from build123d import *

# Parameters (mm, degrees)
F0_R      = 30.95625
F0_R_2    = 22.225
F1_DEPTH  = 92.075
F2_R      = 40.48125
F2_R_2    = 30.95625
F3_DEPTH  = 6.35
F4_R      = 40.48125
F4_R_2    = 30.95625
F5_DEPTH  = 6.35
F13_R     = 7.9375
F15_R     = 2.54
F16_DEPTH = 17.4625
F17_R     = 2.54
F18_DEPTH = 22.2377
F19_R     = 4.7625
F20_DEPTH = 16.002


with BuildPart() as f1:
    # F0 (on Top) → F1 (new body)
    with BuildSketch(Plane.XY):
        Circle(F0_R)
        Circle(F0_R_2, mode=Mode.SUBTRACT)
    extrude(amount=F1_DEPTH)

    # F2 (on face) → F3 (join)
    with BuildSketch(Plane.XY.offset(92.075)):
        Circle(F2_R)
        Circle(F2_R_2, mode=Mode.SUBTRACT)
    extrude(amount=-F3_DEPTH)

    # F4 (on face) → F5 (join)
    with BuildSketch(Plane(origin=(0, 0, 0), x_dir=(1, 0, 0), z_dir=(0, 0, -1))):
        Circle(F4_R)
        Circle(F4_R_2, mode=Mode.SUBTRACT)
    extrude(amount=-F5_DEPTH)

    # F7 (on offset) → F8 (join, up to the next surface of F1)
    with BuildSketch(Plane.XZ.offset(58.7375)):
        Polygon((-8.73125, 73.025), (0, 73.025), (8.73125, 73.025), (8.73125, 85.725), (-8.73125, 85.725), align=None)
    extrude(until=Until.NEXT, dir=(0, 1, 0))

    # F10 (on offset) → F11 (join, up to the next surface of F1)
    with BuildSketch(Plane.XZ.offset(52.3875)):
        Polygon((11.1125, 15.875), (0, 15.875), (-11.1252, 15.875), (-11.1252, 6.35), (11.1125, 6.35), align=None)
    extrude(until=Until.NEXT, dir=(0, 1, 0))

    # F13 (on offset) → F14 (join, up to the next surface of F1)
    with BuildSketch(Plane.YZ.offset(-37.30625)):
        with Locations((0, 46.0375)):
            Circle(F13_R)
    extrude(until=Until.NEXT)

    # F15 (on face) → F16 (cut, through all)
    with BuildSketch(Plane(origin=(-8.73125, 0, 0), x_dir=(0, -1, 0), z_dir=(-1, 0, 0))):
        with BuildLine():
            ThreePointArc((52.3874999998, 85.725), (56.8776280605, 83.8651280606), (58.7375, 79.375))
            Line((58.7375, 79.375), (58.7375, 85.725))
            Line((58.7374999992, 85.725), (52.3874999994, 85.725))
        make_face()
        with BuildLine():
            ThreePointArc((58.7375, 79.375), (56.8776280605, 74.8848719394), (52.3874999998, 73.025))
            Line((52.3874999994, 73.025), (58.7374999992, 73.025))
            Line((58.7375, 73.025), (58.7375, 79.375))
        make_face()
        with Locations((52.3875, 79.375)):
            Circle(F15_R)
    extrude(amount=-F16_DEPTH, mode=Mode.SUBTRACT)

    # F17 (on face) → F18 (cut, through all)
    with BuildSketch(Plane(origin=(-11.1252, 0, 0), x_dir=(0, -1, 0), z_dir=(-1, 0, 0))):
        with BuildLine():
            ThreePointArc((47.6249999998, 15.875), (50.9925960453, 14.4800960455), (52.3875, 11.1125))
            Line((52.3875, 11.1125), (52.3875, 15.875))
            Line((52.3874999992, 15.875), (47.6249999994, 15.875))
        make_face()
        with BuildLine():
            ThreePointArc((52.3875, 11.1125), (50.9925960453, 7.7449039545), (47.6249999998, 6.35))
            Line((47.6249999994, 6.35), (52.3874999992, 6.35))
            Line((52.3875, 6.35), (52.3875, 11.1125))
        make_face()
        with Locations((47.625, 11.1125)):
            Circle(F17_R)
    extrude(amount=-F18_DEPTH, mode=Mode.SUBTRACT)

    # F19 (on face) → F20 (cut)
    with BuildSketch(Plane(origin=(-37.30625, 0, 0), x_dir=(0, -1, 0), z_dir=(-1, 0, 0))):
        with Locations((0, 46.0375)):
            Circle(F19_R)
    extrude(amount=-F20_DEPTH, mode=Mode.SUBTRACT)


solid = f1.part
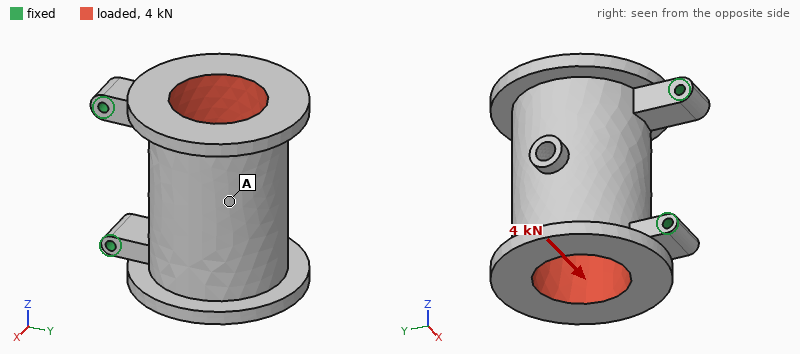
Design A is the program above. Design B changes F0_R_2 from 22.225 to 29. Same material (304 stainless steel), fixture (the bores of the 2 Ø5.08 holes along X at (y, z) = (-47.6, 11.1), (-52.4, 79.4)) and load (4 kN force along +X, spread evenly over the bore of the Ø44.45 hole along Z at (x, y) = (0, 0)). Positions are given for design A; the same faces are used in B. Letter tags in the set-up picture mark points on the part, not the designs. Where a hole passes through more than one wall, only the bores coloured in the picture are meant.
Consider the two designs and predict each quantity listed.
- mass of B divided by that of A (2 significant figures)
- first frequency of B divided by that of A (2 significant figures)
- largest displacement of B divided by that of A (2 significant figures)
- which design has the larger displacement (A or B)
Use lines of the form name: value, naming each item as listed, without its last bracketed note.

mass of B divided by that of A: 0.42
first frequency of B divided by that of A: 0.96
largest displacement of B divided by that of A: 2.6
which design has the larger displacement: B
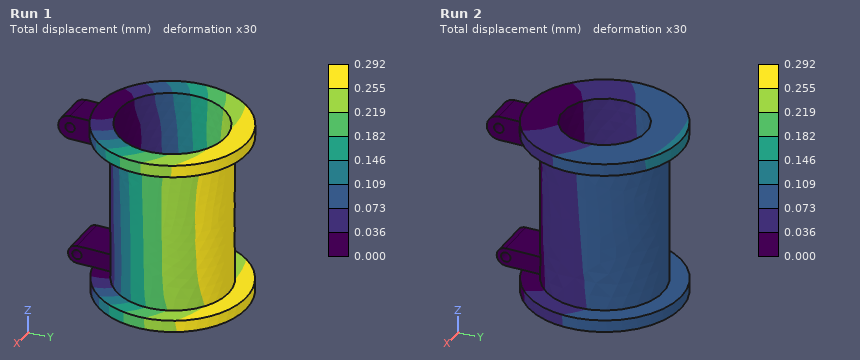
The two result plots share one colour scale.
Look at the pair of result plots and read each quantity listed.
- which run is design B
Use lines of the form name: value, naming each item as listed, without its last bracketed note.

which run is design B: Run 1
